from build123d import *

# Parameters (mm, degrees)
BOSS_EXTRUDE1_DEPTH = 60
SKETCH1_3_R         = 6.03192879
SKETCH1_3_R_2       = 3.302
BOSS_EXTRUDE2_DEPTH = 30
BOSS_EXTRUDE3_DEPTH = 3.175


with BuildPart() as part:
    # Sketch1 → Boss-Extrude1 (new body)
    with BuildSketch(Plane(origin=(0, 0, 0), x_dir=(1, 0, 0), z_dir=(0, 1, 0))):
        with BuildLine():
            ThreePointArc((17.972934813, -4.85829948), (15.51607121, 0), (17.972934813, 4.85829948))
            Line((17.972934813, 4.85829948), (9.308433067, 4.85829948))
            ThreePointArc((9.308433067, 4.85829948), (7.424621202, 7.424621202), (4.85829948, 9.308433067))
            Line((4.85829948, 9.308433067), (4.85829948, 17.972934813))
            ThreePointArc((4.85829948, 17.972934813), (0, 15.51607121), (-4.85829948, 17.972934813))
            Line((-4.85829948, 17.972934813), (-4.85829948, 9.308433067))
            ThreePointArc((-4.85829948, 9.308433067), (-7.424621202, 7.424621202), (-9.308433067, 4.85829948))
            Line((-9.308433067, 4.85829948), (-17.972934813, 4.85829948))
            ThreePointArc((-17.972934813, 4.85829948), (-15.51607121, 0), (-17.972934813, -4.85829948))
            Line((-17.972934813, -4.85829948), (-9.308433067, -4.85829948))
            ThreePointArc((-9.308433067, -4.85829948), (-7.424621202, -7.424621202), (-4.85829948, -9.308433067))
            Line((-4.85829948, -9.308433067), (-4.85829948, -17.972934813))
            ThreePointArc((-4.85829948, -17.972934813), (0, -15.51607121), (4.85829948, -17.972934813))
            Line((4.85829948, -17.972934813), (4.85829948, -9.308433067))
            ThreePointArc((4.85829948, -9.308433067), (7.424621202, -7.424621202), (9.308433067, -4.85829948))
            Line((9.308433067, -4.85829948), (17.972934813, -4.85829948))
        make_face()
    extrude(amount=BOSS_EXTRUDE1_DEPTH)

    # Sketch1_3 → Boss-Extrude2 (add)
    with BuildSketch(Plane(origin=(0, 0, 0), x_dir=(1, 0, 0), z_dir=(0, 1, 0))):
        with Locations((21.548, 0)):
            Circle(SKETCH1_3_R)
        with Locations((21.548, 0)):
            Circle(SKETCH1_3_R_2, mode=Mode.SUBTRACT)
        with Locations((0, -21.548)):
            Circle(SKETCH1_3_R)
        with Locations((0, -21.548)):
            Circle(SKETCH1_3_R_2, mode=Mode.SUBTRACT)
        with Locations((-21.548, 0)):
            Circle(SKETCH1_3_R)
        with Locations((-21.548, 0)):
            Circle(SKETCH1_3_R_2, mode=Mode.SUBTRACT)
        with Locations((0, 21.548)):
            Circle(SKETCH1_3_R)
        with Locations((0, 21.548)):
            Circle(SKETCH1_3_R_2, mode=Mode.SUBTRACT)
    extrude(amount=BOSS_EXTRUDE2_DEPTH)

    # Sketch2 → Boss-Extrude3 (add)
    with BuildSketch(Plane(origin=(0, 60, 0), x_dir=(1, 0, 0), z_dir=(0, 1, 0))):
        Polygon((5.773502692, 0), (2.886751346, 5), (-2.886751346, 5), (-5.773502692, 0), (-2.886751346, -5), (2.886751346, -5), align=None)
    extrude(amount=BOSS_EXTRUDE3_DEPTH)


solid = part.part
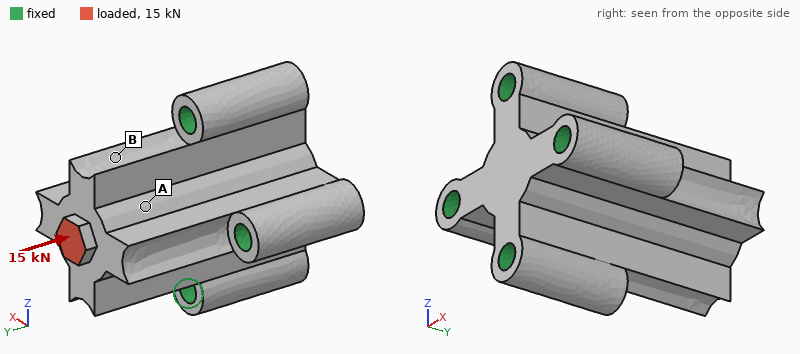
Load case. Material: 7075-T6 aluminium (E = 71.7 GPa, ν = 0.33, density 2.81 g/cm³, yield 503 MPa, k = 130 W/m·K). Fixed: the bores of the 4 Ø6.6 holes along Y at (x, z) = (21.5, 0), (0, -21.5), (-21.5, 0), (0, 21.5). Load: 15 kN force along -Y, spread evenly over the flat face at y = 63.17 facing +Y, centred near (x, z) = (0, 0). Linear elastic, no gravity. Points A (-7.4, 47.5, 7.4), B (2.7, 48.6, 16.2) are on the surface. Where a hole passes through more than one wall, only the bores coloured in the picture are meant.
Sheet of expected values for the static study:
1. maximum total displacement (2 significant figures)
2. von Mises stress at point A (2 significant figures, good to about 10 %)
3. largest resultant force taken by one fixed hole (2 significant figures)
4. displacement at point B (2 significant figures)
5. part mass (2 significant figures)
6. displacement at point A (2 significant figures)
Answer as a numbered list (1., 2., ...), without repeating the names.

1. 33 µm
2. 30 MPa
3. 4.1 kN
4. 11 µm
5. 130 g
6. 12 µm
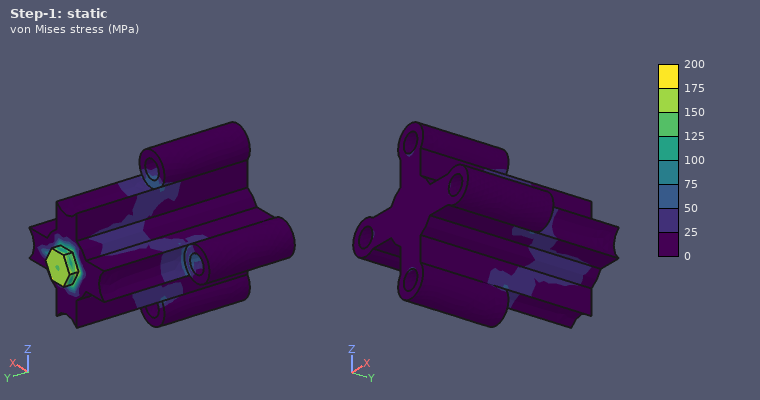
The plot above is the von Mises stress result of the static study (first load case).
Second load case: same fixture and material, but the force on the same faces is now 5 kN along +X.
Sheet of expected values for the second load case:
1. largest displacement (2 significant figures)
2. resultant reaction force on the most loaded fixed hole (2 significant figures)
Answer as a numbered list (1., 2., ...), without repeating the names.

1. 79 µm
2. 5.4 kN
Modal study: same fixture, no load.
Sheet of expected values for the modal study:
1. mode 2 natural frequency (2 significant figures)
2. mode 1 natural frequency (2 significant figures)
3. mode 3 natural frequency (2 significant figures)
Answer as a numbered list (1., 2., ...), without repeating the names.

1. 12 kHz
2. 12 kHz
3. 16 kHz
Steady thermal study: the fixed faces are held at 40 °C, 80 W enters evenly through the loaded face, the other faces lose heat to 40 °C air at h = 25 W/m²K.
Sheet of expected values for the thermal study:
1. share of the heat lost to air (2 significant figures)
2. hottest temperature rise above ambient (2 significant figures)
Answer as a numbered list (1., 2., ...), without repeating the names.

1. 4.2 %
2. 79 K
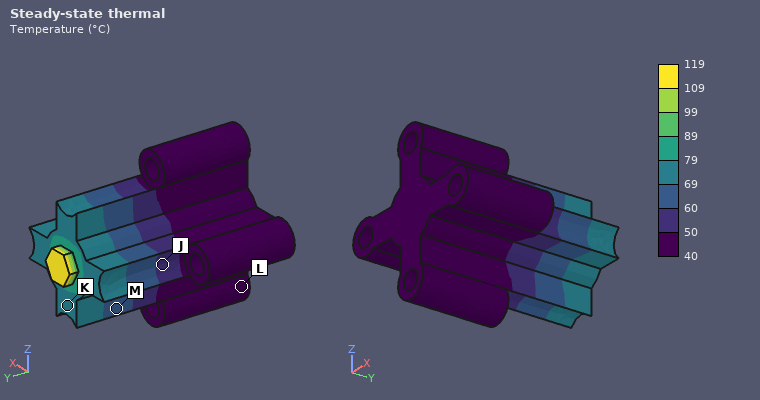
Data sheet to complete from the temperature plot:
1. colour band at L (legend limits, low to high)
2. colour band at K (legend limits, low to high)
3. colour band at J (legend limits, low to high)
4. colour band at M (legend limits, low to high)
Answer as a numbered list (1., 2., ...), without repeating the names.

1. 40 to 50 °C
2. 69 to 79 °C
3. 50 to 60 °C
4. 60 to 69 °C
